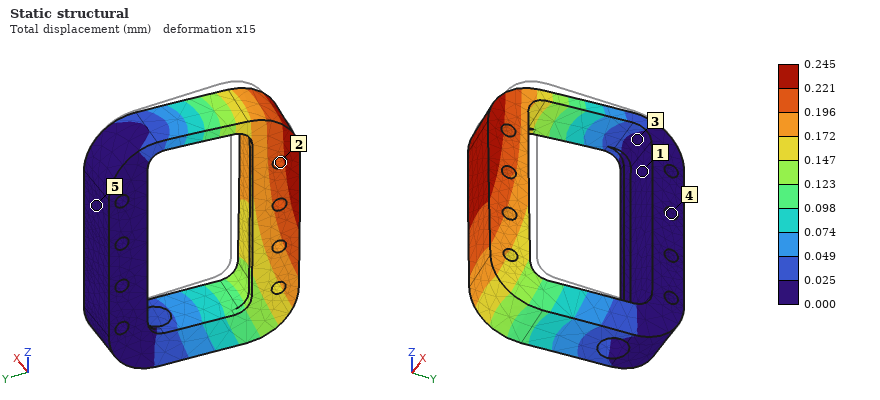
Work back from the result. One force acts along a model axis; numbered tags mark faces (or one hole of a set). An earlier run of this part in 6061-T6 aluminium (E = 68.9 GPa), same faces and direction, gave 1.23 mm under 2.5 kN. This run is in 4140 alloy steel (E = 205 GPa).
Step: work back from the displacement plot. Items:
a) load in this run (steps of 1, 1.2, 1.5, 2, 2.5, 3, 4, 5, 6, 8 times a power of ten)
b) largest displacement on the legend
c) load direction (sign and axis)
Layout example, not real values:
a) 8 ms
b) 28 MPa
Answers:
a) 1.5 kN
b) 0.245 mm
c) -X
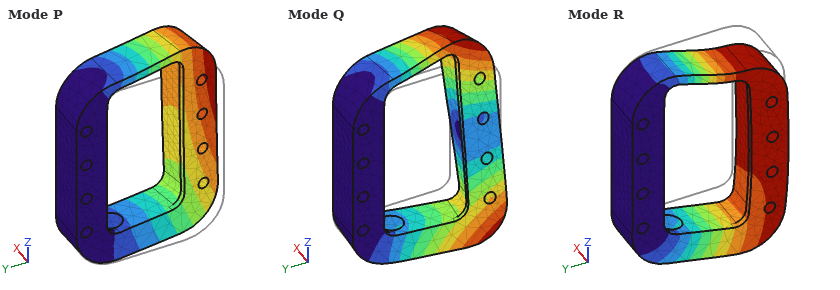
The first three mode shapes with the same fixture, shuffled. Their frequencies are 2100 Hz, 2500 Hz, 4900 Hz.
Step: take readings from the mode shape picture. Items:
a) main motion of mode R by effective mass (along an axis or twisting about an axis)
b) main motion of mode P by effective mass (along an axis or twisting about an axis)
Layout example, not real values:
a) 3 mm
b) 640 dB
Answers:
a) along Z
b) along X
